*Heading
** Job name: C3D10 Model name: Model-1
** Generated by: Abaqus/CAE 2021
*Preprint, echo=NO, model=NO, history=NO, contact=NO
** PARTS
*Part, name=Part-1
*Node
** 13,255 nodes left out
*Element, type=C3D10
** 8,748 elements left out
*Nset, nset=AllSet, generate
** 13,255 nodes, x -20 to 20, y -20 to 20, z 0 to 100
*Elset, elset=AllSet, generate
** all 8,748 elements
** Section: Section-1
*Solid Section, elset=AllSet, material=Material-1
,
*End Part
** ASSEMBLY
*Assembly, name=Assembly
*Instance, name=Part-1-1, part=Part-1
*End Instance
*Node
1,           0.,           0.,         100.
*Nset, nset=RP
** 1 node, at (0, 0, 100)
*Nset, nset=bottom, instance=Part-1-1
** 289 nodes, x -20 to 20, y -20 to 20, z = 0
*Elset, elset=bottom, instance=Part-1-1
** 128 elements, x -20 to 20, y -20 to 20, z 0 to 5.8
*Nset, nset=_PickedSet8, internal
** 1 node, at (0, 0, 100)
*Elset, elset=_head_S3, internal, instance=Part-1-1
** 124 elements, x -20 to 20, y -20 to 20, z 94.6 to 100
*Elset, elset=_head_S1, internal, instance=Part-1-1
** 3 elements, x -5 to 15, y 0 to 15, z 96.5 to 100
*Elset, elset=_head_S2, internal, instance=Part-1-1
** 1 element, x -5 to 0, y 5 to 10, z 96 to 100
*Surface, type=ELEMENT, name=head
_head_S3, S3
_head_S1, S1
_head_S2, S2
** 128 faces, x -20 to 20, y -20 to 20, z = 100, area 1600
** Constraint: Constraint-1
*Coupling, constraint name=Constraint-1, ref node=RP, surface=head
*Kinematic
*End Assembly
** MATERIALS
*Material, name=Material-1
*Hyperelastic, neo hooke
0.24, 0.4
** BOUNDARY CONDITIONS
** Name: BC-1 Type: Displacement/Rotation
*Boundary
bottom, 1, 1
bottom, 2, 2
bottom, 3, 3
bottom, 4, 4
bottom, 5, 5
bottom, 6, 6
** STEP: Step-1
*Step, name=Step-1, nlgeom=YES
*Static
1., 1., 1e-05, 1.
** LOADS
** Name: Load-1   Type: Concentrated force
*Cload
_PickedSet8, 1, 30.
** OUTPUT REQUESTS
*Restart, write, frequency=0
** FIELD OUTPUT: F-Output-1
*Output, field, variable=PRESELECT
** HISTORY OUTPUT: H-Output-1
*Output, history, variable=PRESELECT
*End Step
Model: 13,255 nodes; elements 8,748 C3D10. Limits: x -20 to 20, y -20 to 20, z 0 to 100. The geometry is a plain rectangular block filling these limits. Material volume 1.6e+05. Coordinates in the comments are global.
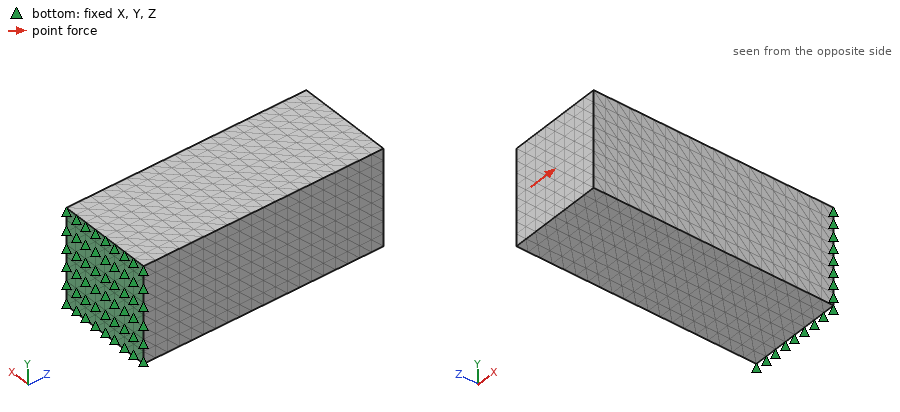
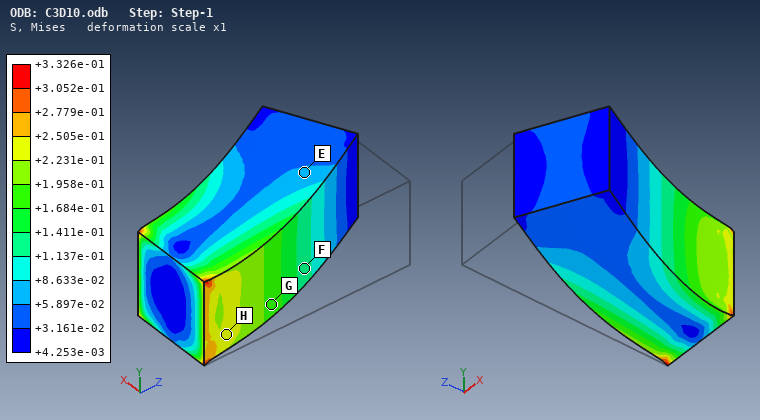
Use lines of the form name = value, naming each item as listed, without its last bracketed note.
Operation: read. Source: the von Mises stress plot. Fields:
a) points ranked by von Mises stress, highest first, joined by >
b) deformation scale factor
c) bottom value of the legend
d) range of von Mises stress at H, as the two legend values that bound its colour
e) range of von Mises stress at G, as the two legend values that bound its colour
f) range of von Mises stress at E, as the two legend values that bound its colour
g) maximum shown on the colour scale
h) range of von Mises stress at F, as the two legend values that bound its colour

points ranked by von Mises stress, highest first, joined by > = H > G > F > E
deformation scale factor = 1
bottom value of the legend = +4.253e-03
range of von Mises stress at H, as the two legend values that bound its colour = +2.231e-01 to +2.505e-01
range of von Mises stress at G, as the two legend values that bound its colour = +1.684e-01 to +1.958e-01
range of von Mises stress at E, as the two legend values that bound its colour = +5.897e-02 to +8.633e-02
maximum shown on the colour scale = +3.326e-01
range of von Mises stress at F, as the two legend values that bound its colour = +1.137e-01 to +1.411e-01
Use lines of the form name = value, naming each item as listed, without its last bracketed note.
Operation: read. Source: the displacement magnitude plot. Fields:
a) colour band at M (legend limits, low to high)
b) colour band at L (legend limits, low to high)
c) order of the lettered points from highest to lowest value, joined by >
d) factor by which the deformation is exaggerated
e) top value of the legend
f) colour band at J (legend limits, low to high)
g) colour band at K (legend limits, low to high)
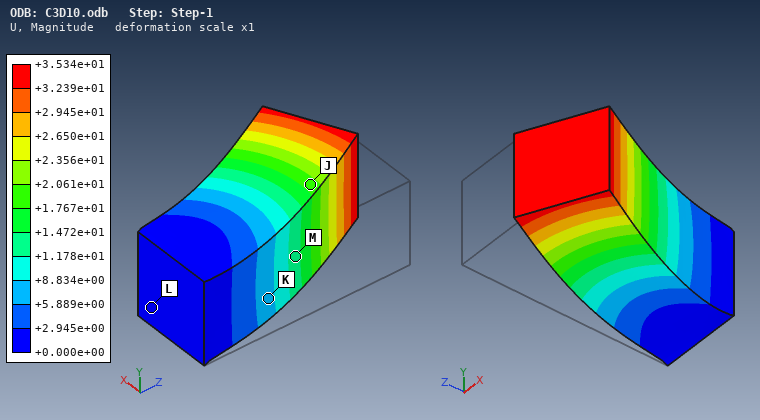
colour band at M = +1.178e+01 to +1.472e+01
colour band at L = +0.000e+00 to +2.945e+00
order of the lettered points from highest to lowest value, joined by > = J > M > K > L
factor by which the deformation is exaggerated = 1
top value of the legend = +3.534e+01
colour band at J = +1.767e+01 to +2.061e+01
colour band at K = +5.889e+00 to +8.834e+00
